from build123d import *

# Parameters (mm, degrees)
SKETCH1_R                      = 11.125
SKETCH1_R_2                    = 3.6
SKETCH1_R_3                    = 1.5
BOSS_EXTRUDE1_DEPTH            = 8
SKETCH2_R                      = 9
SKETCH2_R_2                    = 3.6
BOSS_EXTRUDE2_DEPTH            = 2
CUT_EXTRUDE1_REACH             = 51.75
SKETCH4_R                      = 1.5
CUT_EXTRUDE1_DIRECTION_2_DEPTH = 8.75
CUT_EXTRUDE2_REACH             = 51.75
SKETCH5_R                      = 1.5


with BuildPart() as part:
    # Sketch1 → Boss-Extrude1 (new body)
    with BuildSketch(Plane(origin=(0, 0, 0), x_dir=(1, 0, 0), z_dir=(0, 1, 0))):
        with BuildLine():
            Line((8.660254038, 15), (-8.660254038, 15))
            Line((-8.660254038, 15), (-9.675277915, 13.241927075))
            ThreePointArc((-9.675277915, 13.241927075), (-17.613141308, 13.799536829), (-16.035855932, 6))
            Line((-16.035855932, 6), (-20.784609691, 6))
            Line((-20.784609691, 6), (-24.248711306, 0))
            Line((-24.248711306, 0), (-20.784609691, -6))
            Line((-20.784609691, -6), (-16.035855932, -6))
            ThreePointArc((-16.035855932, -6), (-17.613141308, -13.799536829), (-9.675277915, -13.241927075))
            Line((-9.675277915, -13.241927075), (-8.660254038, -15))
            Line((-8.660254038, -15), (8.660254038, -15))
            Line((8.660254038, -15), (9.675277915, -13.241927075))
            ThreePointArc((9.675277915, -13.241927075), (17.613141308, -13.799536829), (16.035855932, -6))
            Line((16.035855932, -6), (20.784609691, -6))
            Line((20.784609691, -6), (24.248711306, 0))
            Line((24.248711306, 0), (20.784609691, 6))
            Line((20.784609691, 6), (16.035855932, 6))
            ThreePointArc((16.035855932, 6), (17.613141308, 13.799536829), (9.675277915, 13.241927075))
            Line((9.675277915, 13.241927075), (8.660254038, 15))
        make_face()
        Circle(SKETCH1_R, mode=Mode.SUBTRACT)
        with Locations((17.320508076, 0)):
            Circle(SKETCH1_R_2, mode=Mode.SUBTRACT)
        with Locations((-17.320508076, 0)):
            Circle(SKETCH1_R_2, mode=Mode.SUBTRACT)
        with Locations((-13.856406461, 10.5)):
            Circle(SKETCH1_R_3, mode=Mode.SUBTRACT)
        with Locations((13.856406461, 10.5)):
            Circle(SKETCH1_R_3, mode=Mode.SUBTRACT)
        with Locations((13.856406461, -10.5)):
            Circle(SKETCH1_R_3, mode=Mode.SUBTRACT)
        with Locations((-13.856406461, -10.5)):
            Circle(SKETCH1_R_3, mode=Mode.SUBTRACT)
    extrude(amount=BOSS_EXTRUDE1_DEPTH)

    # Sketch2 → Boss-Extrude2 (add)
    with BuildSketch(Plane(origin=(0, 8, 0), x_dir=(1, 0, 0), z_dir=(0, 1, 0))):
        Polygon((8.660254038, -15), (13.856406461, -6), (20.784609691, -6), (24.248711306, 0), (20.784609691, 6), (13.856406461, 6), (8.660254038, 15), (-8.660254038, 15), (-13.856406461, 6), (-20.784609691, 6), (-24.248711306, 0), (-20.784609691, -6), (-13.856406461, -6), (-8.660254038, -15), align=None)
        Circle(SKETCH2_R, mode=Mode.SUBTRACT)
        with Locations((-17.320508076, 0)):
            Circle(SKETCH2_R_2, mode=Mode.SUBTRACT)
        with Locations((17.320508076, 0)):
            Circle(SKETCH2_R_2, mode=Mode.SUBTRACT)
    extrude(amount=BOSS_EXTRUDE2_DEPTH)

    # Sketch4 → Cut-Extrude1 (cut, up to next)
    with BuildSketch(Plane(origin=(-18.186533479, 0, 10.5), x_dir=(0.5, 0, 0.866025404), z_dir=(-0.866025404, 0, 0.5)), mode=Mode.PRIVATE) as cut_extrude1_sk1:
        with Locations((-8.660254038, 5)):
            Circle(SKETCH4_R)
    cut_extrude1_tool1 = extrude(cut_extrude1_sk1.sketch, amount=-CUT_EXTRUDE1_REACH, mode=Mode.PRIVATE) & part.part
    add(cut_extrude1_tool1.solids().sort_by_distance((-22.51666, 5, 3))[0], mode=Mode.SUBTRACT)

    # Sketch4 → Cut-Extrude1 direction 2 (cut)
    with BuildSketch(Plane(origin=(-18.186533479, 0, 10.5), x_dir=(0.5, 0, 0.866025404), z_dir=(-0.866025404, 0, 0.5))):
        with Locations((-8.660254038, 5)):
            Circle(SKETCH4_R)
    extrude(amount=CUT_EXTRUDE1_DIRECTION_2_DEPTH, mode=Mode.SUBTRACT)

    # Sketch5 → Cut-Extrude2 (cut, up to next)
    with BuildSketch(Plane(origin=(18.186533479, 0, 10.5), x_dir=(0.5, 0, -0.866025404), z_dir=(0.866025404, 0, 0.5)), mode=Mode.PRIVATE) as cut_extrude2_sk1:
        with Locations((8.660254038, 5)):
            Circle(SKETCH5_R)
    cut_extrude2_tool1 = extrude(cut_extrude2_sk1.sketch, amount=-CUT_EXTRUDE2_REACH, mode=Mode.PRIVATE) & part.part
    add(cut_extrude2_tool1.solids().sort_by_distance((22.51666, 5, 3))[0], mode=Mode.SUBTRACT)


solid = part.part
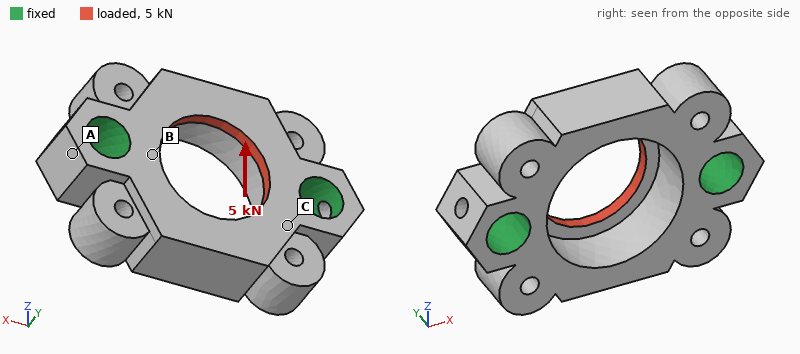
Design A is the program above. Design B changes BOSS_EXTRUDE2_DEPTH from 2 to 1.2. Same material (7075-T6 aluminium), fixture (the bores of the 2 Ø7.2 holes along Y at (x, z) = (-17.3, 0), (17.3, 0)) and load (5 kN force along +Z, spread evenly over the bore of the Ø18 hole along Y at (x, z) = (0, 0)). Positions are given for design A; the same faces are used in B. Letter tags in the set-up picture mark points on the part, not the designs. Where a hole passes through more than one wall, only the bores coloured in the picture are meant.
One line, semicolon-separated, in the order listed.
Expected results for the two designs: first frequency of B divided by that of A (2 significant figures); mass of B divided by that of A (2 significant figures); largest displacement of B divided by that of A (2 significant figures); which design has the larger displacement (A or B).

0.96; 0.93; 1.2; B
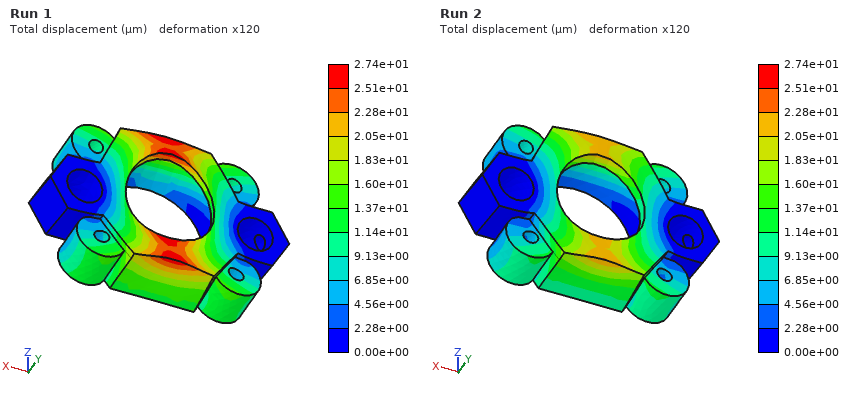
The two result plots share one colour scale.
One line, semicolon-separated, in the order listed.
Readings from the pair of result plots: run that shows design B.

Run 1
